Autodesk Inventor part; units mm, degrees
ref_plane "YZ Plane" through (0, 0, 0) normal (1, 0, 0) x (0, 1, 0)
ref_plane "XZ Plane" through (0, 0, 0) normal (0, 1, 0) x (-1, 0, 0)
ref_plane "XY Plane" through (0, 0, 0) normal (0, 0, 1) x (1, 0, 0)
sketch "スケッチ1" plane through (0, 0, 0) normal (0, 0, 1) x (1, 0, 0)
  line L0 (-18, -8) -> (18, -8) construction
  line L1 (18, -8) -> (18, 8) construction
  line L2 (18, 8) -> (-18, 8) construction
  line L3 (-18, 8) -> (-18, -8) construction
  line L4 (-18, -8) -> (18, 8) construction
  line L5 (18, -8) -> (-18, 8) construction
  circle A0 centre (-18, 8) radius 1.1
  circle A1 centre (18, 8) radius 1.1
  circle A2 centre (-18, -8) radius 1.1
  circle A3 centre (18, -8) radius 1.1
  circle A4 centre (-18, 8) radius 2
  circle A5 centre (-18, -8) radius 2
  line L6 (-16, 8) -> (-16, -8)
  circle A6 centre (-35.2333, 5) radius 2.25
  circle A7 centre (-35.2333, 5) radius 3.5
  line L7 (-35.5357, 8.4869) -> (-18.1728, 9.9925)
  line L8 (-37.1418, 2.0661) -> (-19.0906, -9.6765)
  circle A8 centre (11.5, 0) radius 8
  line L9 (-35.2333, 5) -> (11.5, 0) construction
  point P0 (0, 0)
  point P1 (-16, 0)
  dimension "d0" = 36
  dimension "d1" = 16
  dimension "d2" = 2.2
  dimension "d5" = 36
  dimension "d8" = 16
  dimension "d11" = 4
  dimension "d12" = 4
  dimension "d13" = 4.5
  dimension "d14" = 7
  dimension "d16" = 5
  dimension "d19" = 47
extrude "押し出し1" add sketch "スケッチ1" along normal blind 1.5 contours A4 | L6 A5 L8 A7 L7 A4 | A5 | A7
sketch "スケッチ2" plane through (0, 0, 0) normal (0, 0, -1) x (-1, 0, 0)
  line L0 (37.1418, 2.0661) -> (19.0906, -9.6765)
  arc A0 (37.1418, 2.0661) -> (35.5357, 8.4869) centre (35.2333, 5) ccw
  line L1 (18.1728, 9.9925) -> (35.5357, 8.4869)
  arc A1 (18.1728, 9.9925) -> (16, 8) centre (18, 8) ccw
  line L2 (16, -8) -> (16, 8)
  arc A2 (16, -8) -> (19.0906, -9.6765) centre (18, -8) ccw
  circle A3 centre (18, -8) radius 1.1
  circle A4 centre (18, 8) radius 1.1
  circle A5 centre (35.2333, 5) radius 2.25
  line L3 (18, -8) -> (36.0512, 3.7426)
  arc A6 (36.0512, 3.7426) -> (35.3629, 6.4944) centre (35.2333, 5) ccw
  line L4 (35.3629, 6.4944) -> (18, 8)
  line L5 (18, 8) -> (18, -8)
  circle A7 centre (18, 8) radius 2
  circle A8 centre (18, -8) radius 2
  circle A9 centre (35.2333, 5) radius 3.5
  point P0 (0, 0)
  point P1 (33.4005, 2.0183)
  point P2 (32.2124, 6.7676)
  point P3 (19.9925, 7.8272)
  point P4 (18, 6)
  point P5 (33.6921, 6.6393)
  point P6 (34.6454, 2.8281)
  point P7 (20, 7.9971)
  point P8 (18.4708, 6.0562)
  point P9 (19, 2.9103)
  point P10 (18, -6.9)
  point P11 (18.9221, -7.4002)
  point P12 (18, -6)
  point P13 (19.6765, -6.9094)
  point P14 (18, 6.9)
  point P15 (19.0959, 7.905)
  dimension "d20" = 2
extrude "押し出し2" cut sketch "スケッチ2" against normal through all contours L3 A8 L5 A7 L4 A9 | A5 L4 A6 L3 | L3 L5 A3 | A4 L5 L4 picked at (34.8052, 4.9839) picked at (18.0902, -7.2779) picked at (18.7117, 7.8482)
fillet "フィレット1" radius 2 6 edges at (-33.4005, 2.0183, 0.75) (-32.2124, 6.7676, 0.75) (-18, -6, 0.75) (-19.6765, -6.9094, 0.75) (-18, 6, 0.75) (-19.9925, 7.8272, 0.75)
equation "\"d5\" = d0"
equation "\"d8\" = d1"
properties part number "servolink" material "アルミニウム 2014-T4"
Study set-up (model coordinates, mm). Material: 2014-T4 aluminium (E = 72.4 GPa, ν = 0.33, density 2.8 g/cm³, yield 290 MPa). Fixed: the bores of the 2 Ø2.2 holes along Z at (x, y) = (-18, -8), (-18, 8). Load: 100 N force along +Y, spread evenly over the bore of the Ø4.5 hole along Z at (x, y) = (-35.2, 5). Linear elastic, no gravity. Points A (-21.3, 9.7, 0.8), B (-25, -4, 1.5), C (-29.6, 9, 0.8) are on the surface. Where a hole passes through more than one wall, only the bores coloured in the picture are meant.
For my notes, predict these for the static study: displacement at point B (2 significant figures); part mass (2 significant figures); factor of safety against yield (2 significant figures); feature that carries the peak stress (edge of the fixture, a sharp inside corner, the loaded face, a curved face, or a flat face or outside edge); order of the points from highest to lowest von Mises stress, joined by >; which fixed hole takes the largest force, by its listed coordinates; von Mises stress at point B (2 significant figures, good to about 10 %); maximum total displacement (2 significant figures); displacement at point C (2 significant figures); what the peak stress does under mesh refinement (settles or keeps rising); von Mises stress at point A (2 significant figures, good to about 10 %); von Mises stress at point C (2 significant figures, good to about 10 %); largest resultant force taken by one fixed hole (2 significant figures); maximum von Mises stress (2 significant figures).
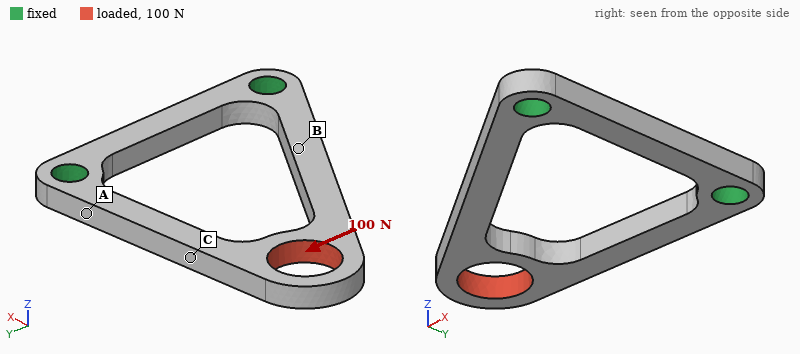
25 µm
0.55 g
1.5
a curved face
A > C > B
(-18, -8)
29 MPa
62 µm
54 µm
settles
130 MPa
84 MPa
100 N
190 MPa
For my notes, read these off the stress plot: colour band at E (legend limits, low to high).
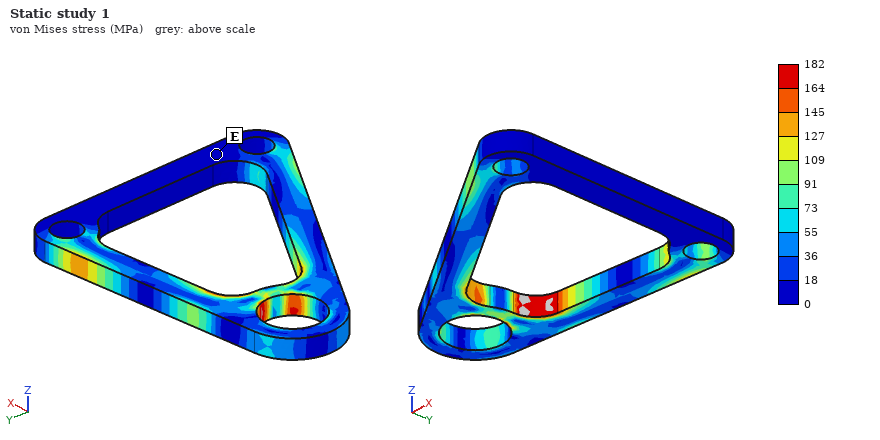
0 to 18 MPa
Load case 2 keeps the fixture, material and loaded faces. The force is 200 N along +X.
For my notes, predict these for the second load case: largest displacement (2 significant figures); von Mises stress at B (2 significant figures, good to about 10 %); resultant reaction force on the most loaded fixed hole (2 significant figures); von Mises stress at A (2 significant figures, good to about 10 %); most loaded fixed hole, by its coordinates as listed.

32 µm
27 MPa
150 N
96 MPa
(-18, 8)
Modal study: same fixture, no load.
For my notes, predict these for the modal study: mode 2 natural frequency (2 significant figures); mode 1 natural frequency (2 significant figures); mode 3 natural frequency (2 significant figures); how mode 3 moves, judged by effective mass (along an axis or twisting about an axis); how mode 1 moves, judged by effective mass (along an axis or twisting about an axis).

11 kHz
2900 Hz
13 kHz
along Y
along Z
